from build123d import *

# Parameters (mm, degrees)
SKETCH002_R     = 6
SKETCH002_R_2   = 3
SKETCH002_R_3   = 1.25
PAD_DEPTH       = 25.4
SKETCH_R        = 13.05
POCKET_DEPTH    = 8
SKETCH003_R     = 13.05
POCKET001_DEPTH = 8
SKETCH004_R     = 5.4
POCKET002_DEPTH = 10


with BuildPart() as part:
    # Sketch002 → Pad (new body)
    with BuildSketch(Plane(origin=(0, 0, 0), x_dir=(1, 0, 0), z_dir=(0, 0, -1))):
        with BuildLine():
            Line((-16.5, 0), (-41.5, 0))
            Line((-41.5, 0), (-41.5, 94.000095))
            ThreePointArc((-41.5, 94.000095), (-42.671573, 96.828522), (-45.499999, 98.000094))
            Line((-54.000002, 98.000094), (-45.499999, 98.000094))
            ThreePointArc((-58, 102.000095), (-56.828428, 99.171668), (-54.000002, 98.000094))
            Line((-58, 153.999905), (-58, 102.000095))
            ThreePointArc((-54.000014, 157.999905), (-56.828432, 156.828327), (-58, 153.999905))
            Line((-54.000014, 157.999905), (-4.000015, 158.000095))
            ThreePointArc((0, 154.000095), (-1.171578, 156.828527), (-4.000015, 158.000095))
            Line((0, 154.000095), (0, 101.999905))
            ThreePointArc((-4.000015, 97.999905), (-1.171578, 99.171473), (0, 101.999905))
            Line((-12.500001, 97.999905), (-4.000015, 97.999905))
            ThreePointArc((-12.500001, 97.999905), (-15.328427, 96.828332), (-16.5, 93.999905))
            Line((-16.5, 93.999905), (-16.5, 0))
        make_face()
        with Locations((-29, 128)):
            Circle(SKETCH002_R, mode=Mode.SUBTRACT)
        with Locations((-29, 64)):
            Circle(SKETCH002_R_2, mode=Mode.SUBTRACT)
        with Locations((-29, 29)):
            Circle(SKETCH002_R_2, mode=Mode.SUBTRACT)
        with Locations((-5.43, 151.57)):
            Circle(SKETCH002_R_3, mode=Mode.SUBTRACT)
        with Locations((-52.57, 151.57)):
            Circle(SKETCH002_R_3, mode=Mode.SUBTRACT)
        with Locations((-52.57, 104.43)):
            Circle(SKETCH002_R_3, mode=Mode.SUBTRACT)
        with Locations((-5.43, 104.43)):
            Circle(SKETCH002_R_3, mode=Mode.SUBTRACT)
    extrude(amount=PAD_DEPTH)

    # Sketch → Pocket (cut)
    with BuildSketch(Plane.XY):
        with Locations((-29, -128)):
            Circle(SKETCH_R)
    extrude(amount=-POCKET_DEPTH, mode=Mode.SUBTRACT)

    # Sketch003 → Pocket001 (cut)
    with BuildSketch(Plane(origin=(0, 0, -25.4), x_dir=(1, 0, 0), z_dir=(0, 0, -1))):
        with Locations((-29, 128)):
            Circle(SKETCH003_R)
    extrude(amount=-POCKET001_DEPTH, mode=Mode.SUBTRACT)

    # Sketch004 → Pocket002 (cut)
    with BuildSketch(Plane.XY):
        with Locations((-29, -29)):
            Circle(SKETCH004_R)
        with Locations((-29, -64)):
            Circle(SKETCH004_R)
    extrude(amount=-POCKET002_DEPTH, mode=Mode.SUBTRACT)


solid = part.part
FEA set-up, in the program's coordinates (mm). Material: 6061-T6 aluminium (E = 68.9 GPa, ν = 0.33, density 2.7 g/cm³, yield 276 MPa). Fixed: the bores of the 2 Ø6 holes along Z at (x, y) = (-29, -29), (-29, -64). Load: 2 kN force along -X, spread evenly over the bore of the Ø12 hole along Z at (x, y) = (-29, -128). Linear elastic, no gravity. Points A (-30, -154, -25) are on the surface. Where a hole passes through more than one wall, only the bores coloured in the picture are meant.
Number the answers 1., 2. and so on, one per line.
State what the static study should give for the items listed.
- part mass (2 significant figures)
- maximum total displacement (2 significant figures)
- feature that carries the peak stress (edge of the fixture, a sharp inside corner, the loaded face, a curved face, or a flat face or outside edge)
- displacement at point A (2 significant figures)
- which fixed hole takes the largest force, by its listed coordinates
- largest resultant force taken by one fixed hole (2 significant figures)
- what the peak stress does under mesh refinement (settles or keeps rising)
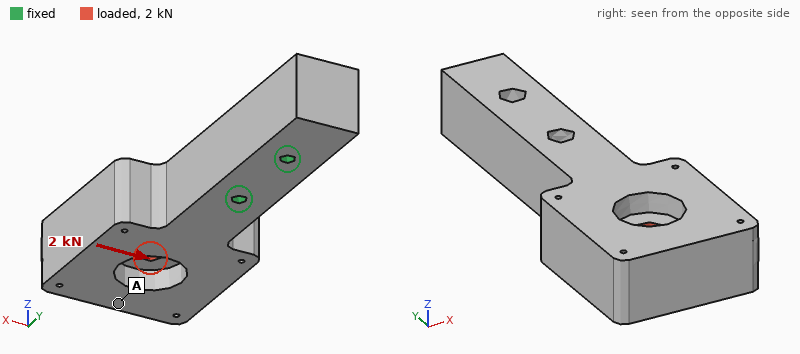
1. 370 g
2. 0.21 mm
3. edge of the fixture
4. 0.19 mm
5. (-29, -64)
6. 4.6 kN
7. keeps rising
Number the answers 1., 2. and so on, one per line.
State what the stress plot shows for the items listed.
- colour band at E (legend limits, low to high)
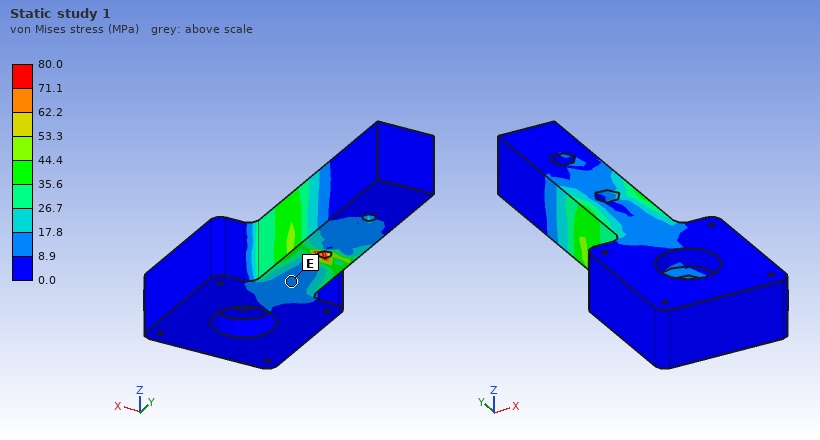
1. 8.9 to 17.8 MPa
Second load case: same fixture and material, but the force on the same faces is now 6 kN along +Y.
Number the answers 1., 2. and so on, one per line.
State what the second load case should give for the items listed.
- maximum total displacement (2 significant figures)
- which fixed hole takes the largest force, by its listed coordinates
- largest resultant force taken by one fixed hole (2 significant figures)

1. 21 µm
2. (-29, -64)
3. 4.8 kN
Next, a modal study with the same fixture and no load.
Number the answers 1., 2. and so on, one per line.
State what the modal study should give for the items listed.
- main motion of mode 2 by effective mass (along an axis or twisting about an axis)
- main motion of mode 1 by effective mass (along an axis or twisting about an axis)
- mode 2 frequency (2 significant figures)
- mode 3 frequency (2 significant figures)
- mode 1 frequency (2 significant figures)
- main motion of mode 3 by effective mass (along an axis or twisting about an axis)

1. along Z
2. along X
3. 1300 Hz
4. 3000 Hz
5. 1200 Hz
6. twisting about Y
